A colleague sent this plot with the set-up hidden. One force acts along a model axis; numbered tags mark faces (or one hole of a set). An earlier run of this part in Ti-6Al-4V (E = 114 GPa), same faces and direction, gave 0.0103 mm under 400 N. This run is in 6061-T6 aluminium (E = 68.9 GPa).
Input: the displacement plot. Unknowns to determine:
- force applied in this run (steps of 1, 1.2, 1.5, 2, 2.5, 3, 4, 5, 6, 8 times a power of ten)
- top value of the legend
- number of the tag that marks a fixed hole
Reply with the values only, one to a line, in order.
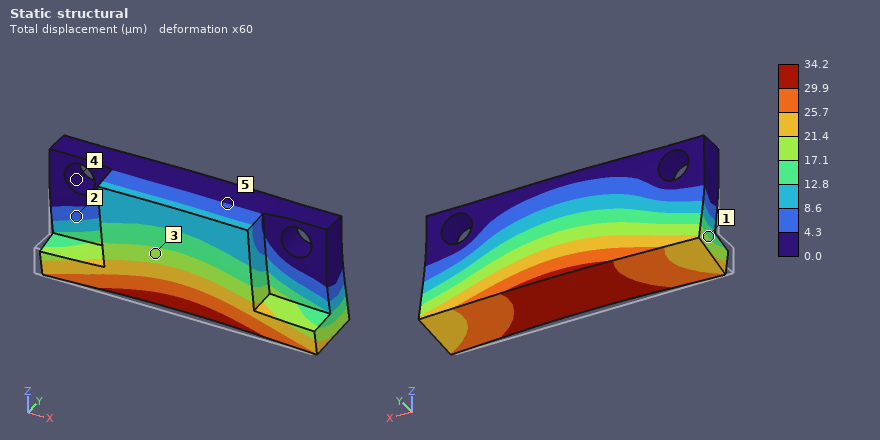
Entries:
800 N
34.2 µm
4
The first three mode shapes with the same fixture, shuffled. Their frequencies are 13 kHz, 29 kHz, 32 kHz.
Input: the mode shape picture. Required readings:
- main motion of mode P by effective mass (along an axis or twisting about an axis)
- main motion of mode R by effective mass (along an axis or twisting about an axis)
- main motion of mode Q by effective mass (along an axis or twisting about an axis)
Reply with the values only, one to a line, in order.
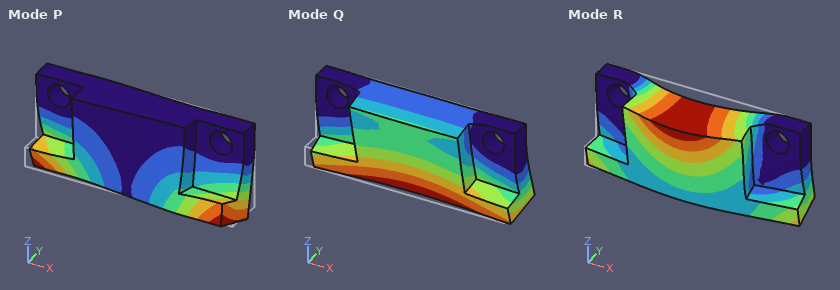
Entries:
twisting about Z
along Y
along Y
